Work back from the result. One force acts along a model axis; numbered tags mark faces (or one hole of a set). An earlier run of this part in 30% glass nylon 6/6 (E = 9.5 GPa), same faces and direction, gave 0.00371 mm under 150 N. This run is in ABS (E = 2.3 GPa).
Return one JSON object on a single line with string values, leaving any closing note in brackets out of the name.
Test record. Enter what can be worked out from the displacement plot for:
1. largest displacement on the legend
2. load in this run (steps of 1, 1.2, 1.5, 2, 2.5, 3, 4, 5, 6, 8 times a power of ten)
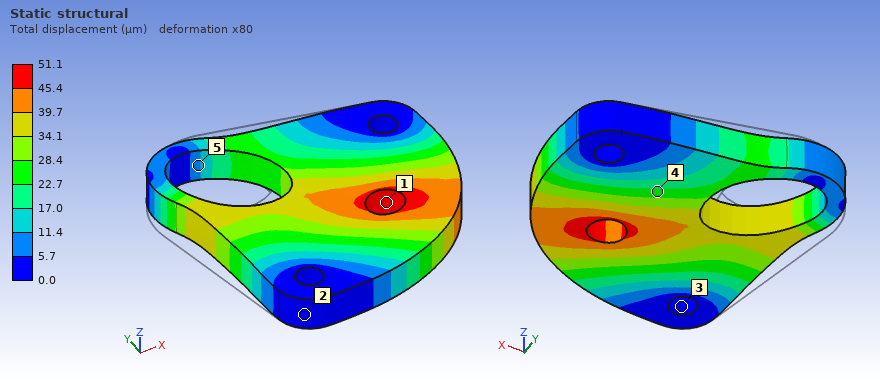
{"largest displacement on the legend": "51.1 µm", "load in this run": "500 N"}
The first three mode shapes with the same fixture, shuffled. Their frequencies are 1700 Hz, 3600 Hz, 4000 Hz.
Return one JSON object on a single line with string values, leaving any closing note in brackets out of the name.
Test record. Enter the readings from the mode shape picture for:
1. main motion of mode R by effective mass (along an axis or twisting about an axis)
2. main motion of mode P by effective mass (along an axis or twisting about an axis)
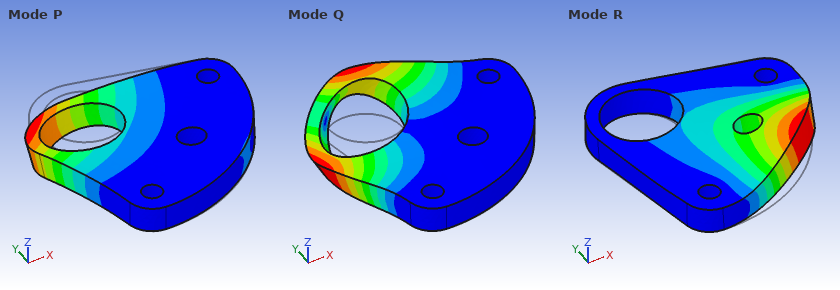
{"main motion of mode R by effective mass": "along Z", "main motion of mode P by effective mass": "along Z"}
